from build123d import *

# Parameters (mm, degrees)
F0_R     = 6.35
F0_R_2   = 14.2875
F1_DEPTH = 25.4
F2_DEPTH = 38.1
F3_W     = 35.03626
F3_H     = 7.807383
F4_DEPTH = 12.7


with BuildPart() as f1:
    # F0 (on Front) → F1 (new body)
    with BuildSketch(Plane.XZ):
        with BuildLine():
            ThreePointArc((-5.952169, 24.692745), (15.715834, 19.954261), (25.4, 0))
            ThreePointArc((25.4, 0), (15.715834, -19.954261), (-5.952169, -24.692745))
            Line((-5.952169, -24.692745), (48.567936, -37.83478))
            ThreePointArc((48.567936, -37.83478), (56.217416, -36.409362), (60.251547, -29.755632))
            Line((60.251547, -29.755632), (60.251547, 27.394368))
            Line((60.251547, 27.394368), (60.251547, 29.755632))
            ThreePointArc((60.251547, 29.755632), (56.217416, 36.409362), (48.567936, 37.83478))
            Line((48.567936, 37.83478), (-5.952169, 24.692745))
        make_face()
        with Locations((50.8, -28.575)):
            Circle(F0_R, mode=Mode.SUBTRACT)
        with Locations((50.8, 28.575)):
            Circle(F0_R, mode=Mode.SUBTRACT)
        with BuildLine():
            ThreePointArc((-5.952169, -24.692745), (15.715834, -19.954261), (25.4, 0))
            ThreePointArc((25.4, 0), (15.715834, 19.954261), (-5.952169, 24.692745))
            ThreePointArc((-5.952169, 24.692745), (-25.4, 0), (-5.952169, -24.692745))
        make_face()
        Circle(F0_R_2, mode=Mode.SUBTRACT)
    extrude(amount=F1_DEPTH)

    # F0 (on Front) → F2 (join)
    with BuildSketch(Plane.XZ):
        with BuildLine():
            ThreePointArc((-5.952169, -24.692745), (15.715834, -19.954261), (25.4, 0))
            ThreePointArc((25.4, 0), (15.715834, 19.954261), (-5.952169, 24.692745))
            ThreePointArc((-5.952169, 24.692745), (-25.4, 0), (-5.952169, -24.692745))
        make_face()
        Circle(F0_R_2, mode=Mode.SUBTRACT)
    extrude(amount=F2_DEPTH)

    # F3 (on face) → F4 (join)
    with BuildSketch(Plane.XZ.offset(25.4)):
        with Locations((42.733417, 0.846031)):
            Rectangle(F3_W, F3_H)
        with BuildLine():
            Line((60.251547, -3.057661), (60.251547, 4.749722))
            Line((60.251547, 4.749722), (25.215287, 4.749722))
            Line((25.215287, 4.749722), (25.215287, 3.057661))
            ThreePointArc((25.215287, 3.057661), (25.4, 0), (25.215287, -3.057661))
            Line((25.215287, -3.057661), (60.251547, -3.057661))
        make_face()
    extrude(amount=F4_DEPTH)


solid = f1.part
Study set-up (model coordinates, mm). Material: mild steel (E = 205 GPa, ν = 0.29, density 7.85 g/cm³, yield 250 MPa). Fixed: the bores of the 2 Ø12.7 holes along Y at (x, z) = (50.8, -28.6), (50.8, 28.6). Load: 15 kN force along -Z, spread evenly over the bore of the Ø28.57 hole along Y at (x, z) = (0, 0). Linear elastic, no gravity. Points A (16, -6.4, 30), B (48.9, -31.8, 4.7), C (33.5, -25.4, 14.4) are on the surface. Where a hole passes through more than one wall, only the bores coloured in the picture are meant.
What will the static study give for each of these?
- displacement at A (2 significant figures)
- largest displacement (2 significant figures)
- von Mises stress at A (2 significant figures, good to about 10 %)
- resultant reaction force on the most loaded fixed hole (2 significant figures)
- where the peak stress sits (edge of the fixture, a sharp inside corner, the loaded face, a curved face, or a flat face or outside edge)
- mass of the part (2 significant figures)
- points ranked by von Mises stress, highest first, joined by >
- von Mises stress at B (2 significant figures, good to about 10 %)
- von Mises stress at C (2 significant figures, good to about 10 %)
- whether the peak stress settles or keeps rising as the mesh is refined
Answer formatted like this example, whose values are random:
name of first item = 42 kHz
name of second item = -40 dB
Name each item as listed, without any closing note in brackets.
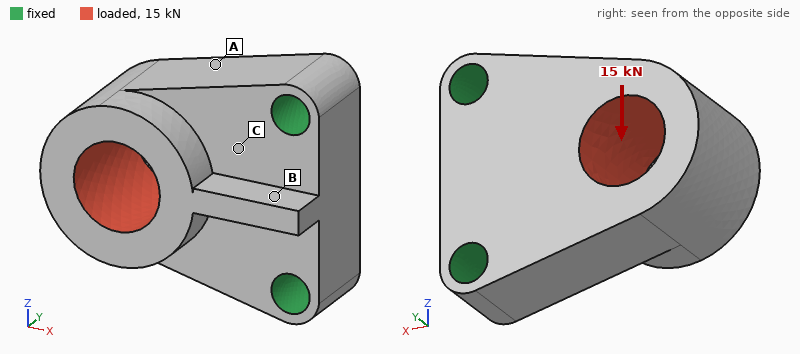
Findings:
displacement at A = 6.8 µm
largest displacement = 21 µm
von Mises stress at A = 32 MPa
resultant reaction force on the most loaded fixed hole = 15 kN
where the peak stress sits = edge of the fixture
mass of the part = 980 g
points ranked by von Mises stress, highest first, joined by > = A > C > B
von Mises stress at B = 7.1 MPa
von Mises stress at C = 22 MPa
whether the peak stress settles or keeps rising as the mesh is refined = keeps rising
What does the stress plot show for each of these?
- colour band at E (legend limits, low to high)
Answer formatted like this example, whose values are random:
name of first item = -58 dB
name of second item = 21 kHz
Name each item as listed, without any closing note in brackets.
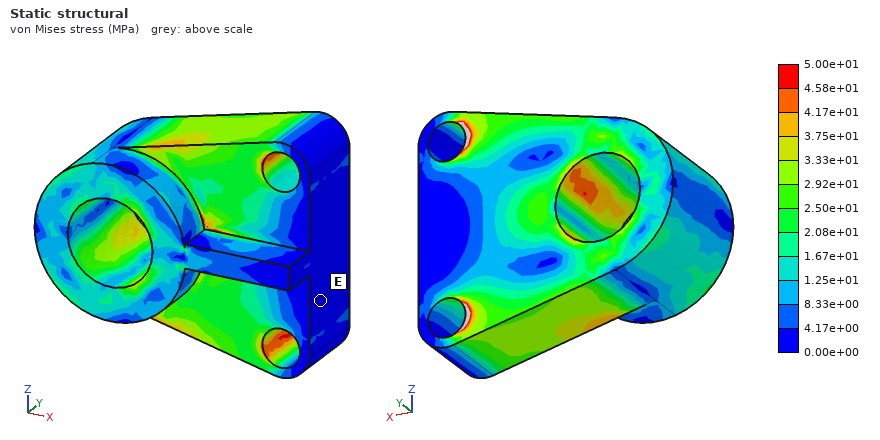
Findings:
colour band at E = 0.00e+00 to 4.17e+00 MPa
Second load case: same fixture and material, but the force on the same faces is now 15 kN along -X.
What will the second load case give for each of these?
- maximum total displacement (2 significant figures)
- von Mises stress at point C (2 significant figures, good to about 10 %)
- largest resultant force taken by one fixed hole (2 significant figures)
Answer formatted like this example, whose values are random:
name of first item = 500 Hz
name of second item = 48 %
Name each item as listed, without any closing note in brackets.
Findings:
maximum total displacement = 16 µm
von Mises stress at point C = 18 MPa
largest resultant force taken by one fixed hole = 7.8 kN
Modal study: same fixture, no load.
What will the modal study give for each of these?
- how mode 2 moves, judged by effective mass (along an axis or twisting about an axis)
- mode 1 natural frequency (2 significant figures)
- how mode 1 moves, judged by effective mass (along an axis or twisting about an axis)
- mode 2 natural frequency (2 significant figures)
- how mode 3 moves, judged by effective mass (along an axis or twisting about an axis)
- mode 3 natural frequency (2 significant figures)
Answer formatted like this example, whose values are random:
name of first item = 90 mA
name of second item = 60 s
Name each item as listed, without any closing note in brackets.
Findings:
how mode 2 moves, judged by effective mass = along Z
mode 1 natural frequency = 3800 Hz
how mode 1 moves, judged by effective mass = along Y
mode 2 natural frequency = 7400 Hz
how mode 3 moves, judged by effective mass = twisting about X
mode 3 natural frequency = 9400 Hz
